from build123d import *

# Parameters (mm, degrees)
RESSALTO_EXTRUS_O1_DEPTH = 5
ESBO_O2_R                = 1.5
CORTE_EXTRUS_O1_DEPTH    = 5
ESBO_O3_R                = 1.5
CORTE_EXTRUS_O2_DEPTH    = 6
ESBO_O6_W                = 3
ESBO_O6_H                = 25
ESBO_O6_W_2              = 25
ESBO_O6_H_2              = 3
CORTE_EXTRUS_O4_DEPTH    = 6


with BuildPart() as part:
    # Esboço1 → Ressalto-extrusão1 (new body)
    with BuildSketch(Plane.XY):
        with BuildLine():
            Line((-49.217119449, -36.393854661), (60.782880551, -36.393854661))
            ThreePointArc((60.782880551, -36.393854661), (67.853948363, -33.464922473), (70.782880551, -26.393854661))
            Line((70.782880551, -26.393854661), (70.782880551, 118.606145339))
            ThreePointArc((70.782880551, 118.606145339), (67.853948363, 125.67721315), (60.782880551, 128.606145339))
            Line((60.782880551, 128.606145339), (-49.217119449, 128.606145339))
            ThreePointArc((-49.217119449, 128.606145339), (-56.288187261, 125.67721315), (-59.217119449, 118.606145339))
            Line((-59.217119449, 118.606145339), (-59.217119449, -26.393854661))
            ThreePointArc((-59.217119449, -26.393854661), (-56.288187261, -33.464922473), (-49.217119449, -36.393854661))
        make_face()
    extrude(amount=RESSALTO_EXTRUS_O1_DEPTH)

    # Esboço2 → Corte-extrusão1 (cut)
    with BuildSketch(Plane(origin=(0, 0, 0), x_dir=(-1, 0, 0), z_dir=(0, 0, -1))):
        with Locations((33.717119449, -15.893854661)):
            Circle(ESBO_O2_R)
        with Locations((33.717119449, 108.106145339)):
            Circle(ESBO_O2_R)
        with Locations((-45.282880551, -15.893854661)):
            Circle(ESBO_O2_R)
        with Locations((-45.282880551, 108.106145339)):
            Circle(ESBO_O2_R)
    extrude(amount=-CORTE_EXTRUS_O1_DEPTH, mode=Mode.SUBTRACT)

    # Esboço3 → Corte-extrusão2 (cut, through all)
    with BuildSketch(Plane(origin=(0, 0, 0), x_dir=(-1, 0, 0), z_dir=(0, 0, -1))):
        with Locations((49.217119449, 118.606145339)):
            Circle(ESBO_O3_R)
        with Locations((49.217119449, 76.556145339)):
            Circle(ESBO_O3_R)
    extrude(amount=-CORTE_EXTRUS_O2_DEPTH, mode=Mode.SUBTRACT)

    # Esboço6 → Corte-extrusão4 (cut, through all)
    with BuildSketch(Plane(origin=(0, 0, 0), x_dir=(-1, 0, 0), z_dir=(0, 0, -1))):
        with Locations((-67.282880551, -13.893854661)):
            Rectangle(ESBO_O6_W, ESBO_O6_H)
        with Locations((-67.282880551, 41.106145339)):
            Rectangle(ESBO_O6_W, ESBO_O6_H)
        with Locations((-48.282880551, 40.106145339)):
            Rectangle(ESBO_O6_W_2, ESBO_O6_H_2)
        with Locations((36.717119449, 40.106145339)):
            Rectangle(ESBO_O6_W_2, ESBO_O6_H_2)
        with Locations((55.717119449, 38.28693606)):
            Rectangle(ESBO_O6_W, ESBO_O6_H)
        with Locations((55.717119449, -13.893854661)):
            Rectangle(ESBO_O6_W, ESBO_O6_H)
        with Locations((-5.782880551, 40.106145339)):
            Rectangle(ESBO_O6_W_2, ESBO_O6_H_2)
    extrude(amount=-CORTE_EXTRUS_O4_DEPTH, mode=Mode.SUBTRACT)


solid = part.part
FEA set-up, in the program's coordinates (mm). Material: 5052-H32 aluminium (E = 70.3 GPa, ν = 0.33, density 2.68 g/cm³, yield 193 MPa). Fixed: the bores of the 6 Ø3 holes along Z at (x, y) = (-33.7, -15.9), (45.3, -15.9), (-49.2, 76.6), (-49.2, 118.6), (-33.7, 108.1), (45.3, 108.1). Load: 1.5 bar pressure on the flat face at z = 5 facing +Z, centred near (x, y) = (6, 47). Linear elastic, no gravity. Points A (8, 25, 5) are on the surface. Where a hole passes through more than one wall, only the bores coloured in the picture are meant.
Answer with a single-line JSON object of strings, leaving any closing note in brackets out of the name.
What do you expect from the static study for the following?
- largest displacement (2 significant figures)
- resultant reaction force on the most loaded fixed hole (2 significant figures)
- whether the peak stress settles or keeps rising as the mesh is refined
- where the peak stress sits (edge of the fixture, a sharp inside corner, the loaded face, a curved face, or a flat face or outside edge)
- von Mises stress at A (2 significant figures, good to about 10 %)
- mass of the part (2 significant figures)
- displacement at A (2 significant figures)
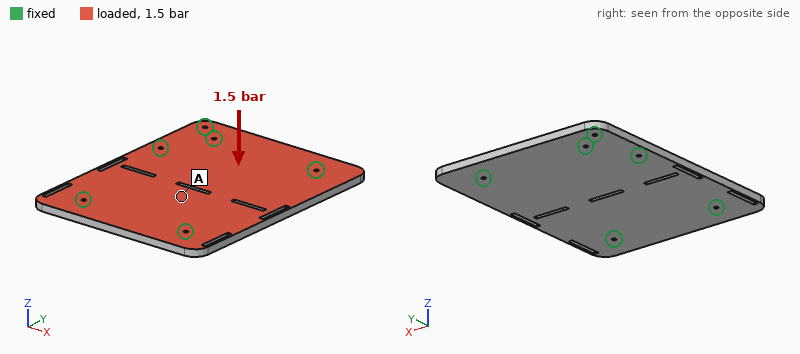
{"largest displacement": "0.23 mm", "resultant reaction force on the most loaded fixed hole": "790 N", "whether the peak stress settles or keeps rising as the mesh is refined": "keeps rising", "where the peak stress sits": "edge of the fixture", "von Mises stress at A": "14 MPa", "mass of the part": "280 g", "displacement at A": "0.16 mm"}
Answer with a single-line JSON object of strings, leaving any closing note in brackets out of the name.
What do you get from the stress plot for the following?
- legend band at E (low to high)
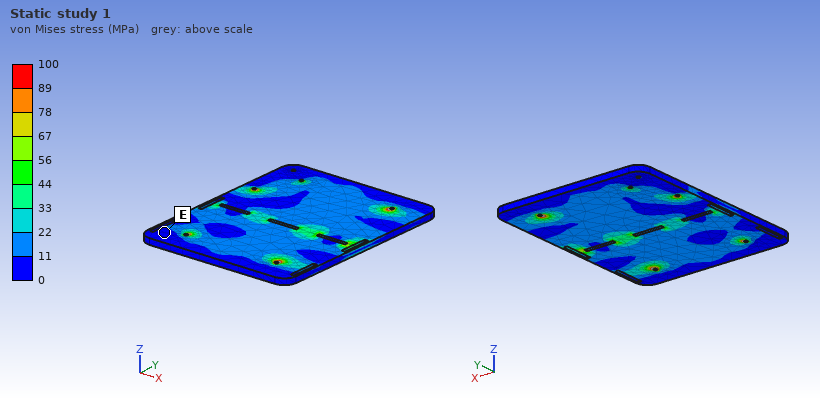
{"legend band at E": "0 to 11 MPa"}
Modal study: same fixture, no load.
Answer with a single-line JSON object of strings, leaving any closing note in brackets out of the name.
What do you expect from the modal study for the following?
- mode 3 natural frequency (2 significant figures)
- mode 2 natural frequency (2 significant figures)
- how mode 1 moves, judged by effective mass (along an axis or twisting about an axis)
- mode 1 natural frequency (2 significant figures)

{"mode 3 natural frequency": "2900 Hz", "mode 2 natural frequency": "2100 Hz", "how mode 1 moves, judged by effective mass": "along Z", "mode 1 natural frequency": "1400 Hz"}
